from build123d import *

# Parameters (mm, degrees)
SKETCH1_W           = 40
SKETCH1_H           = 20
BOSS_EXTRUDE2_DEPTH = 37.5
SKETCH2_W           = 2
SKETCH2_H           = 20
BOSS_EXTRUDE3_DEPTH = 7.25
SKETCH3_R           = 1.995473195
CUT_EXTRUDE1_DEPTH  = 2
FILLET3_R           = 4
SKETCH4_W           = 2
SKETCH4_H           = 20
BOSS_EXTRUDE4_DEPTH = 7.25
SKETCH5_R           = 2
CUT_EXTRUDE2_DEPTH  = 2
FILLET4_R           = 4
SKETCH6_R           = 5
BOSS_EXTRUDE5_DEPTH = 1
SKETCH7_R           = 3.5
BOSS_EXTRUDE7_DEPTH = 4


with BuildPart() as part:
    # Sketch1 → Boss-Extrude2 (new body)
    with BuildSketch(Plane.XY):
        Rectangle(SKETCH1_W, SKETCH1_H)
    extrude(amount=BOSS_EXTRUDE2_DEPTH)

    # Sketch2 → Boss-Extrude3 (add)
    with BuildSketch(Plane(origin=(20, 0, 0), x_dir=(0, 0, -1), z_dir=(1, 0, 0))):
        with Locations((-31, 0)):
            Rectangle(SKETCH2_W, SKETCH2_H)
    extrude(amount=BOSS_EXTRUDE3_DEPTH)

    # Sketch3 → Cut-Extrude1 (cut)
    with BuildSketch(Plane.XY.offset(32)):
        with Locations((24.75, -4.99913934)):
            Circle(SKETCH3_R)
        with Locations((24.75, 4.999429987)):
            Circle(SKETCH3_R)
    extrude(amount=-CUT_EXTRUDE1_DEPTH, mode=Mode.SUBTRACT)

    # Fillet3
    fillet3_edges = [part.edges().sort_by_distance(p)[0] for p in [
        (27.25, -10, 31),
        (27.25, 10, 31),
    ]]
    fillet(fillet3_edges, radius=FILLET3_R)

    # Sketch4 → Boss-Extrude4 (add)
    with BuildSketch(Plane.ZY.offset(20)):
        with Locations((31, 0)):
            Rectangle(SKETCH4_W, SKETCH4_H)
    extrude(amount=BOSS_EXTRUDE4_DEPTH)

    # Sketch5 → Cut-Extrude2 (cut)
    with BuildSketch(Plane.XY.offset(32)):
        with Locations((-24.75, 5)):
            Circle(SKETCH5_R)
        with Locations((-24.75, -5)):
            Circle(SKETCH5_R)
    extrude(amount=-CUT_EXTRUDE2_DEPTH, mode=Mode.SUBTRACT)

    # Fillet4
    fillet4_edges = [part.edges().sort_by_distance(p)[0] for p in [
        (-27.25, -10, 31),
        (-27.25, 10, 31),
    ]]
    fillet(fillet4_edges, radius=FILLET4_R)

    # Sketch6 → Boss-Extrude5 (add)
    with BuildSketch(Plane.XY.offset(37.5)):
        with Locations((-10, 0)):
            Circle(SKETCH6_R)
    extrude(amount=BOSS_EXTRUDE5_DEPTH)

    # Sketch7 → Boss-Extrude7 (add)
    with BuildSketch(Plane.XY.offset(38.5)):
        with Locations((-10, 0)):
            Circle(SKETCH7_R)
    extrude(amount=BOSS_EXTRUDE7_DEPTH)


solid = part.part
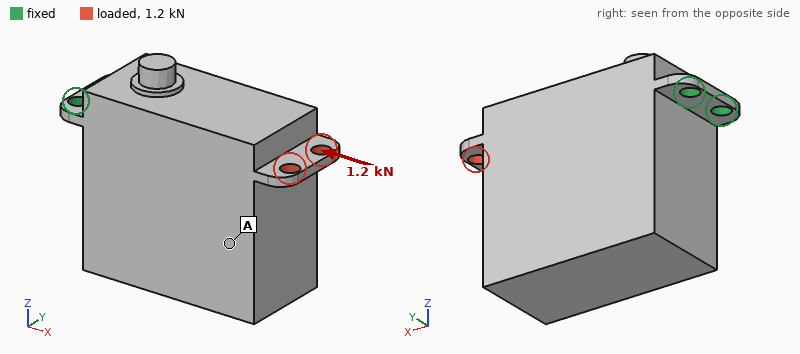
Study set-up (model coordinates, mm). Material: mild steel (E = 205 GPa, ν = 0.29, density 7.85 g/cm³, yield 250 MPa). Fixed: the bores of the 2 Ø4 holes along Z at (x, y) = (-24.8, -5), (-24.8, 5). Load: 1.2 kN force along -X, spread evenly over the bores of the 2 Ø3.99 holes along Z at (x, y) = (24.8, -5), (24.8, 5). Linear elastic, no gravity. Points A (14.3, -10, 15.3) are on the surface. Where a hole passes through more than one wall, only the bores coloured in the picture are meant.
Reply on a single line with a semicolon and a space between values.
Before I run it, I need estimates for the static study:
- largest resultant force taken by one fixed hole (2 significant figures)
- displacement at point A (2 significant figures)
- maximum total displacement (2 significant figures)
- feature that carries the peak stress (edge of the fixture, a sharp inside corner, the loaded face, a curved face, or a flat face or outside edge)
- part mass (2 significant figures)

600 N; 1.2 µm; 5.9 µm; a flat face or outside edge; 240 g
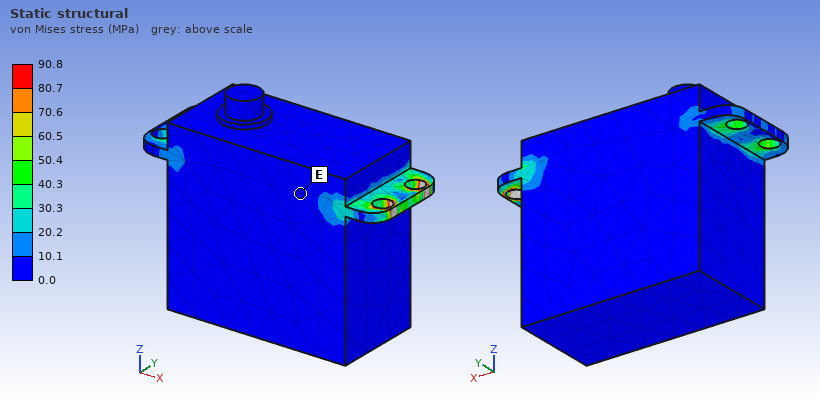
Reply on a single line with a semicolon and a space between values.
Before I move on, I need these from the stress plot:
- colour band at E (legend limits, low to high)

0.0 to 10.1 MPa
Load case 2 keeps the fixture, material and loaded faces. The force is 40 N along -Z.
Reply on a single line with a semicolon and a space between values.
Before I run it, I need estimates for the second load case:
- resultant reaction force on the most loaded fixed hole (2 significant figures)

21 N
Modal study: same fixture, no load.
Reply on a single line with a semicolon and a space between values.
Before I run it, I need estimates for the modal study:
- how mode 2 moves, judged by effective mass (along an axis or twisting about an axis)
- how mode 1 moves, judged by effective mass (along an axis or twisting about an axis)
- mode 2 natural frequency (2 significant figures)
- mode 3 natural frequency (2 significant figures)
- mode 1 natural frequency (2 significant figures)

along Y; along Z; 1500 Hz; 3200 Hz; 290 Hz
